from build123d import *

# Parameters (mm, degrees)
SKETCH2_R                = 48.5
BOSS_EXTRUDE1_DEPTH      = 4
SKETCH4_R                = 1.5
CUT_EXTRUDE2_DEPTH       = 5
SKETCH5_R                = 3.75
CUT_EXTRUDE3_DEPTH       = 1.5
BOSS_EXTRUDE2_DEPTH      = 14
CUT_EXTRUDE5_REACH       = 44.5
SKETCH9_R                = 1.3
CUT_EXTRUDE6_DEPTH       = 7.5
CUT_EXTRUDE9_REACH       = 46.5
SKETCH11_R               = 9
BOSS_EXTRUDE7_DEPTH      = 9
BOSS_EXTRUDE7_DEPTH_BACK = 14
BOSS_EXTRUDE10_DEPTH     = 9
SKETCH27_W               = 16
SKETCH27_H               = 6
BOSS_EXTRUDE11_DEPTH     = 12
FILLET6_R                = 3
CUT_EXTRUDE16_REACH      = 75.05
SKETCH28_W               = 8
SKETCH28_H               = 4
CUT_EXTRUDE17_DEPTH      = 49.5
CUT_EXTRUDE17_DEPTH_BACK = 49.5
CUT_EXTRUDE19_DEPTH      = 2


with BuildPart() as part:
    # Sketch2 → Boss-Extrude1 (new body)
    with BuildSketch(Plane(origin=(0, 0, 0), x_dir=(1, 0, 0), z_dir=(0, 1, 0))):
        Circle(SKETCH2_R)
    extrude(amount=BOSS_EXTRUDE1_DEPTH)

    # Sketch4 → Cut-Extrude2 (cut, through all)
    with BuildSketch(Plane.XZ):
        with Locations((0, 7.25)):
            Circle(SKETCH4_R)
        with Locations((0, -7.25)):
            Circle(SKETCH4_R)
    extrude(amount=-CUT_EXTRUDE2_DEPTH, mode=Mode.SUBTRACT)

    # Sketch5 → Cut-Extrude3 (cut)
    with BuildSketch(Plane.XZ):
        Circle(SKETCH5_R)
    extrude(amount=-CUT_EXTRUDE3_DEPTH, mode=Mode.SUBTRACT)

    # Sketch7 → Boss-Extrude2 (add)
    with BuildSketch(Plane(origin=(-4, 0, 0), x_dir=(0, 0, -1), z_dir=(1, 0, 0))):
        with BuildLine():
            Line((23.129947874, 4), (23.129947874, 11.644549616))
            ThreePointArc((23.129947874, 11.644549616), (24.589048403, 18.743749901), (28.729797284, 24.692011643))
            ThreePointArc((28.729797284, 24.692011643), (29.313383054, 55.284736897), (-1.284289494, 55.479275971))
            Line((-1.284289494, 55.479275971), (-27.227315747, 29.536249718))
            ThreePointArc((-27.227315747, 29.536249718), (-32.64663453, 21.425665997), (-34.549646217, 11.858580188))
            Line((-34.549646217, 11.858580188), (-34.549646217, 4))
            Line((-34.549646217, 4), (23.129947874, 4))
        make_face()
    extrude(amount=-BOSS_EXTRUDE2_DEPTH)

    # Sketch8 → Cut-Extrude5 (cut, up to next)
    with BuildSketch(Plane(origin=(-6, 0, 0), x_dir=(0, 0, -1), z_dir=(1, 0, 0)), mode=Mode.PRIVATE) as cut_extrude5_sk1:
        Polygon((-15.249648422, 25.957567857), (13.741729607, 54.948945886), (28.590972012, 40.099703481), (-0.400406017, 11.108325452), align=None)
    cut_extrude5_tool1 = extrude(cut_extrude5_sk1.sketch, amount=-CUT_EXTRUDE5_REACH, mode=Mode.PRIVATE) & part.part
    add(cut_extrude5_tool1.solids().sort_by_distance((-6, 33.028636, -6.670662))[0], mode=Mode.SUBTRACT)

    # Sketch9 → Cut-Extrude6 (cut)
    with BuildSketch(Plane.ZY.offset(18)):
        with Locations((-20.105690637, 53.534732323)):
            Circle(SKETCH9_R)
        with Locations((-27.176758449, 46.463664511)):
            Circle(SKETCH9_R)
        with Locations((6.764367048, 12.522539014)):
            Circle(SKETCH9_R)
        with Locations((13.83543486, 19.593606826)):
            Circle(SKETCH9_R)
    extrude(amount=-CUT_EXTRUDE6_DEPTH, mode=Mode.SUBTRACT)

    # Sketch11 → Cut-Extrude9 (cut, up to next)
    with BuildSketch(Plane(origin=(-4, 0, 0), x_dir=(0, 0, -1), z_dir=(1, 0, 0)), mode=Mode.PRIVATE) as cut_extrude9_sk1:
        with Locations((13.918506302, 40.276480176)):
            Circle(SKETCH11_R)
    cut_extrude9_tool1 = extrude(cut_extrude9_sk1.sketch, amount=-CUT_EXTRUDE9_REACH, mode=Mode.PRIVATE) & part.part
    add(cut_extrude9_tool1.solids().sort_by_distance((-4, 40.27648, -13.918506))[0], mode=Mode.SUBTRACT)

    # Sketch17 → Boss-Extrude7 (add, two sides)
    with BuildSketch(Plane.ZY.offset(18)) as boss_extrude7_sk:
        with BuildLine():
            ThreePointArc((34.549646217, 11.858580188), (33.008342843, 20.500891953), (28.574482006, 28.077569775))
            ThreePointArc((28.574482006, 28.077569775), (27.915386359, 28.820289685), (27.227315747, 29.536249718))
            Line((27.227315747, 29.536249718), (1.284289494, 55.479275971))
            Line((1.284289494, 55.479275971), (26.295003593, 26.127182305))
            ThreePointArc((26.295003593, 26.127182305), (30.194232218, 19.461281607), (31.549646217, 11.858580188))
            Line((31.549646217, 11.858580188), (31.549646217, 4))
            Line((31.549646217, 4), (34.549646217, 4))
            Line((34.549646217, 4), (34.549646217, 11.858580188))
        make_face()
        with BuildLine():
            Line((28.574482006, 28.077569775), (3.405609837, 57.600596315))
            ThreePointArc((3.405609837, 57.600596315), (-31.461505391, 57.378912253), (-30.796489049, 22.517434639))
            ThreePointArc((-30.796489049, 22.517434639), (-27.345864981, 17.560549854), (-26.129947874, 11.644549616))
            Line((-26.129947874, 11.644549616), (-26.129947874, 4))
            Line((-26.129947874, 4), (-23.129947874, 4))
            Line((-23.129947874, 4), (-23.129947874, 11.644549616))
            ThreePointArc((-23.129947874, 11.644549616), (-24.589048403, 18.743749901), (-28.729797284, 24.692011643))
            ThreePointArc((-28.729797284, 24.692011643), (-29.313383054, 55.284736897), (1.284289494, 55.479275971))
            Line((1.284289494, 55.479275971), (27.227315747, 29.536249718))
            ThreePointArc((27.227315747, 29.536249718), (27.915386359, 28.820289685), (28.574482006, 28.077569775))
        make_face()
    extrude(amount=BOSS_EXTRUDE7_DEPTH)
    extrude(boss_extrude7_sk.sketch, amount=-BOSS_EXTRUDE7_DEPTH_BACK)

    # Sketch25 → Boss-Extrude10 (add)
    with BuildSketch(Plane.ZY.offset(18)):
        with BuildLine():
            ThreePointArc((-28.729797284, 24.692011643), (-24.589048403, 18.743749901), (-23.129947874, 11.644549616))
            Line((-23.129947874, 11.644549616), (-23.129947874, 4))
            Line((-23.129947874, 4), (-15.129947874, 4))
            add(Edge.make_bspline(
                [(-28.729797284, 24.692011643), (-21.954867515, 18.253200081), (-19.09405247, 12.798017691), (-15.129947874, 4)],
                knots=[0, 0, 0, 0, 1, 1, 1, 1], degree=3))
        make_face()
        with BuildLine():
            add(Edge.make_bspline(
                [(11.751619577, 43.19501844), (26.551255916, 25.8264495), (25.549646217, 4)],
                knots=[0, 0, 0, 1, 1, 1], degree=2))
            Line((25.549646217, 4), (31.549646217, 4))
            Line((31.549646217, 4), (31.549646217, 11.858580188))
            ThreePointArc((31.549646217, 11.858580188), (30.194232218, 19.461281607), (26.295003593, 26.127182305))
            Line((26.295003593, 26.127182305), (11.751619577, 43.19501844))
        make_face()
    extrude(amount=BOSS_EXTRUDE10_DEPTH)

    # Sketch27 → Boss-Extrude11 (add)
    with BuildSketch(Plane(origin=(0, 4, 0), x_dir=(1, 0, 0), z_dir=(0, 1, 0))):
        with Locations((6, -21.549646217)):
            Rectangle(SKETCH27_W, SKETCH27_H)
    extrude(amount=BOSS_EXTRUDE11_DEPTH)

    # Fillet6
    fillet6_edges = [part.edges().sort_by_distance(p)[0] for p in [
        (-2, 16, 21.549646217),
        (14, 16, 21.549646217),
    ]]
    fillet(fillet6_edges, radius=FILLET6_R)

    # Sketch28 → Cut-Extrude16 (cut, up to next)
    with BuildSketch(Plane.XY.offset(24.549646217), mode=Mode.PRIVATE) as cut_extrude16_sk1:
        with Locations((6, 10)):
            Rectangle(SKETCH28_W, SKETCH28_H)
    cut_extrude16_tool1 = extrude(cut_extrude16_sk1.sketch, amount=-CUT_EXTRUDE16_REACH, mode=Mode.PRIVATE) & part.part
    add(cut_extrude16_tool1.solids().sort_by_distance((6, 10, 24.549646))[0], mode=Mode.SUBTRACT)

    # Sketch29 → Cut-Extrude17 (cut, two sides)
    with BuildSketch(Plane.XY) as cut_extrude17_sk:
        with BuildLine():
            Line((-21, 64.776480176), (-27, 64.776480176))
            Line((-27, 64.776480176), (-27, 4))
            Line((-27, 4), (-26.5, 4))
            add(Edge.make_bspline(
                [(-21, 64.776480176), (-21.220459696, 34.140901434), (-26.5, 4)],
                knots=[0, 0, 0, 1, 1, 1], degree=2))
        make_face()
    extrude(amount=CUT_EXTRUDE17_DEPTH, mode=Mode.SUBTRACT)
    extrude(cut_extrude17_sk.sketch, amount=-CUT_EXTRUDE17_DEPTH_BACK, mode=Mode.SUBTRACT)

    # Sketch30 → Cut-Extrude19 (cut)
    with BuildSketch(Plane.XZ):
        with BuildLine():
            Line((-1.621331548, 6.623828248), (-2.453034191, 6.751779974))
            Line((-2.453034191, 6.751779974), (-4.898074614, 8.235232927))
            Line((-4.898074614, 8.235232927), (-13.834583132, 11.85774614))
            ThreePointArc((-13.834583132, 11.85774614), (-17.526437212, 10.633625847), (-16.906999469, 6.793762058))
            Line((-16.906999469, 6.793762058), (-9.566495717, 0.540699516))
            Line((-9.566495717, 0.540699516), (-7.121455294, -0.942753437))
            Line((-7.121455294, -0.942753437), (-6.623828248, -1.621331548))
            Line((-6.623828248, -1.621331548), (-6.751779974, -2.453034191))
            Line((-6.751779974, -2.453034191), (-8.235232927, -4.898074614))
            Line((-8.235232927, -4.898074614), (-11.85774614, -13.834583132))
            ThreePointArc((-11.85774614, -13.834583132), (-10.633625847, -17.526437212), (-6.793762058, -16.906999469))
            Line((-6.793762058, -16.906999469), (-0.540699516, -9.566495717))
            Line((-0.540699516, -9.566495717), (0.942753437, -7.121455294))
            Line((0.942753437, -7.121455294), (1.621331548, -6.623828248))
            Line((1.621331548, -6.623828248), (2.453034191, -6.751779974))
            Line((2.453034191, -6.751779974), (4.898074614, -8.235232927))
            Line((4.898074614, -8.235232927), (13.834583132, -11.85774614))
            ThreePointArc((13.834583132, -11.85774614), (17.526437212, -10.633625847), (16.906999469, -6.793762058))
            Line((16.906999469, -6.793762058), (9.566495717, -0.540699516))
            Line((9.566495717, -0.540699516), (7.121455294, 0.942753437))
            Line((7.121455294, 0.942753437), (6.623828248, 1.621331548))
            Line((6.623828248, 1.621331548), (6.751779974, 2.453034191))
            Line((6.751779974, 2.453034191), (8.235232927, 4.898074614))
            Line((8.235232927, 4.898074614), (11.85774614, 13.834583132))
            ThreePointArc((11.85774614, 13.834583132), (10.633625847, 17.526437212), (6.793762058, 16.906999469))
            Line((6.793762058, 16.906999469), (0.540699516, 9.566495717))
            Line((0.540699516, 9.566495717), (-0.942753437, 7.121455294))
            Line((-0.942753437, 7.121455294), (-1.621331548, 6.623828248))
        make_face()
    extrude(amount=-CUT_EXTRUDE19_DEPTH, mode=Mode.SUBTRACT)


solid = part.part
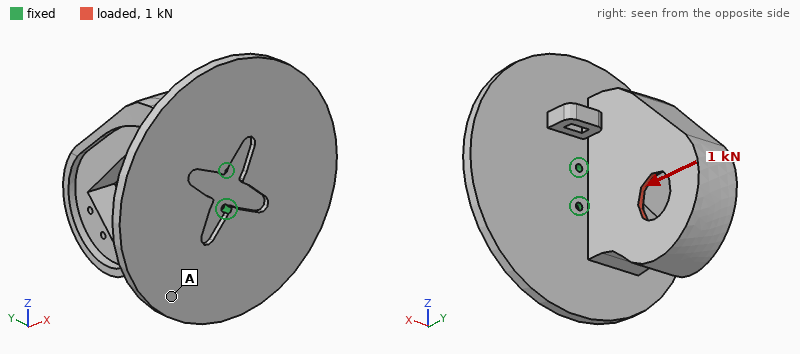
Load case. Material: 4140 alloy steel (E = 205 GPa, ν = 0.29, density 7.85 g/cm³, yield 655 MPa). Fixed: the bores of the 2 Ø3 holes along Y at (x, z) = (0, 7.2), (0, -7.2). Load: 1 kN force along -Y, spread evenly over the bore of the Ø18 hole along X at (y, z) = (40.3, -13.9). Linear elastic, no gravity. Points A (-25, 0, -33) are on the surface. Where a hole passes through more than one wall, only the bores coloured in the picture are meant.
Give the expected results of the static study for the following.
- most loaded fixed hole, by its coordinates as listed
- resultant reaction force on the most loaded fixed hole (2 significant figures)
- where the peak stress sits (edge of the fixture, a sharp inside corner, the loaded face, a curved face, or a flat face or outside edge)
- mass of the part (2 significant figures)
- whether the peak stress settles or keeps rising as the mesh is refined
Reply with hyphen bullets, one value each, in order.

- (0, -7.2)
- 1.2 kN
- edge of the fixture
- 530 g
- keeps rising
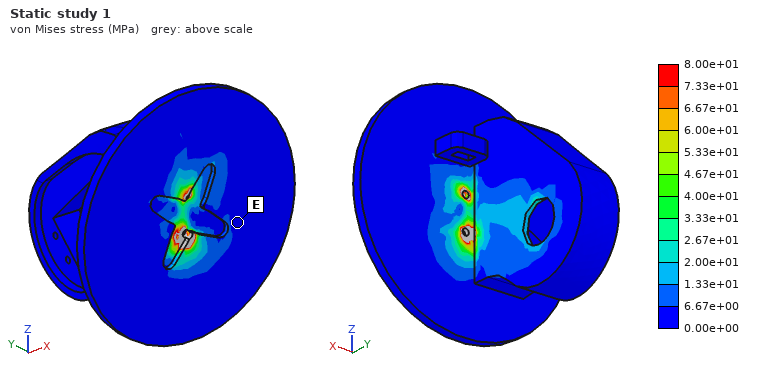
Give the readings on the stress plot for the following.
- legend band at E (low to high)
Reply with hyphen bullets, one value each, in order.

- 0.00e+00 to 6.67e+00 MPa
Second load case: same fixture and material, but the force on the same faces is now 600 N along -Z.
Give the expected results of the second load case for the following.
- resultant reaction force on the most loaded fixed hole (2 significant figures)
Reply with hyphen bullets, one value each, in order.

- 1.2 kN
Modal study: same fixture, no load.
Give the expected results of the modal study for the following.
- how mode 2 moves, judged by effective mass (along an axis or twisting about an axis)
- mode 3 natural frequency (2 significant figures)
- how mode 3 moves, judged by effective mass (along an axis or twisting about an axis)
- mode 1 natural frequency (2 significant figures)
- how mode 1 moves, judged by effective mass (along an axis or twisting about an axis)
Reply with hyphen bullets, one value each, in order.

- along Z
- 1500 Hz
- along Y
- 450 Hz
- along X
